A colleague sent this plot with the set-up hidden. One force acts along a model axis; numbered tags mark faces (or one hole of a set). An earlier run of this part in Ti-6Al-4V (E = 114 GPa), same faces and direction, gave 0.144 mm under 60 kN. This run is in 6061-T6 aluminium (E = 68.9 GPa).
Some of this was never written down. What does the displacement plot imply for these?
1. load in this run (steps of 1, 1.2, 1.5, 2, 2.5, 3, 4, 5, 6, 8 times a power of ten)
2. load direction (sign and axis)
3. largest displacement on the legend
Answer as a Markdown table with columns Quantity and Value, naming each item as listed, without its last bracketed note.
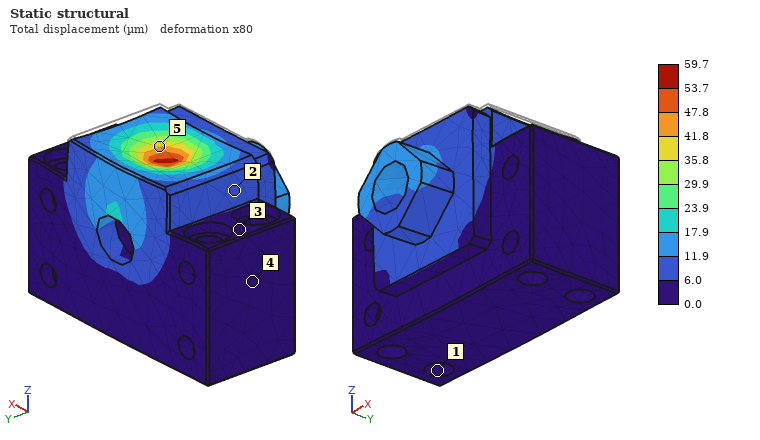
| Quantity | Value |
|---|---|
| load in this run | 15 kN |
| load direction | -Z |
| largest displacement on the legend | 59.7 µm |
